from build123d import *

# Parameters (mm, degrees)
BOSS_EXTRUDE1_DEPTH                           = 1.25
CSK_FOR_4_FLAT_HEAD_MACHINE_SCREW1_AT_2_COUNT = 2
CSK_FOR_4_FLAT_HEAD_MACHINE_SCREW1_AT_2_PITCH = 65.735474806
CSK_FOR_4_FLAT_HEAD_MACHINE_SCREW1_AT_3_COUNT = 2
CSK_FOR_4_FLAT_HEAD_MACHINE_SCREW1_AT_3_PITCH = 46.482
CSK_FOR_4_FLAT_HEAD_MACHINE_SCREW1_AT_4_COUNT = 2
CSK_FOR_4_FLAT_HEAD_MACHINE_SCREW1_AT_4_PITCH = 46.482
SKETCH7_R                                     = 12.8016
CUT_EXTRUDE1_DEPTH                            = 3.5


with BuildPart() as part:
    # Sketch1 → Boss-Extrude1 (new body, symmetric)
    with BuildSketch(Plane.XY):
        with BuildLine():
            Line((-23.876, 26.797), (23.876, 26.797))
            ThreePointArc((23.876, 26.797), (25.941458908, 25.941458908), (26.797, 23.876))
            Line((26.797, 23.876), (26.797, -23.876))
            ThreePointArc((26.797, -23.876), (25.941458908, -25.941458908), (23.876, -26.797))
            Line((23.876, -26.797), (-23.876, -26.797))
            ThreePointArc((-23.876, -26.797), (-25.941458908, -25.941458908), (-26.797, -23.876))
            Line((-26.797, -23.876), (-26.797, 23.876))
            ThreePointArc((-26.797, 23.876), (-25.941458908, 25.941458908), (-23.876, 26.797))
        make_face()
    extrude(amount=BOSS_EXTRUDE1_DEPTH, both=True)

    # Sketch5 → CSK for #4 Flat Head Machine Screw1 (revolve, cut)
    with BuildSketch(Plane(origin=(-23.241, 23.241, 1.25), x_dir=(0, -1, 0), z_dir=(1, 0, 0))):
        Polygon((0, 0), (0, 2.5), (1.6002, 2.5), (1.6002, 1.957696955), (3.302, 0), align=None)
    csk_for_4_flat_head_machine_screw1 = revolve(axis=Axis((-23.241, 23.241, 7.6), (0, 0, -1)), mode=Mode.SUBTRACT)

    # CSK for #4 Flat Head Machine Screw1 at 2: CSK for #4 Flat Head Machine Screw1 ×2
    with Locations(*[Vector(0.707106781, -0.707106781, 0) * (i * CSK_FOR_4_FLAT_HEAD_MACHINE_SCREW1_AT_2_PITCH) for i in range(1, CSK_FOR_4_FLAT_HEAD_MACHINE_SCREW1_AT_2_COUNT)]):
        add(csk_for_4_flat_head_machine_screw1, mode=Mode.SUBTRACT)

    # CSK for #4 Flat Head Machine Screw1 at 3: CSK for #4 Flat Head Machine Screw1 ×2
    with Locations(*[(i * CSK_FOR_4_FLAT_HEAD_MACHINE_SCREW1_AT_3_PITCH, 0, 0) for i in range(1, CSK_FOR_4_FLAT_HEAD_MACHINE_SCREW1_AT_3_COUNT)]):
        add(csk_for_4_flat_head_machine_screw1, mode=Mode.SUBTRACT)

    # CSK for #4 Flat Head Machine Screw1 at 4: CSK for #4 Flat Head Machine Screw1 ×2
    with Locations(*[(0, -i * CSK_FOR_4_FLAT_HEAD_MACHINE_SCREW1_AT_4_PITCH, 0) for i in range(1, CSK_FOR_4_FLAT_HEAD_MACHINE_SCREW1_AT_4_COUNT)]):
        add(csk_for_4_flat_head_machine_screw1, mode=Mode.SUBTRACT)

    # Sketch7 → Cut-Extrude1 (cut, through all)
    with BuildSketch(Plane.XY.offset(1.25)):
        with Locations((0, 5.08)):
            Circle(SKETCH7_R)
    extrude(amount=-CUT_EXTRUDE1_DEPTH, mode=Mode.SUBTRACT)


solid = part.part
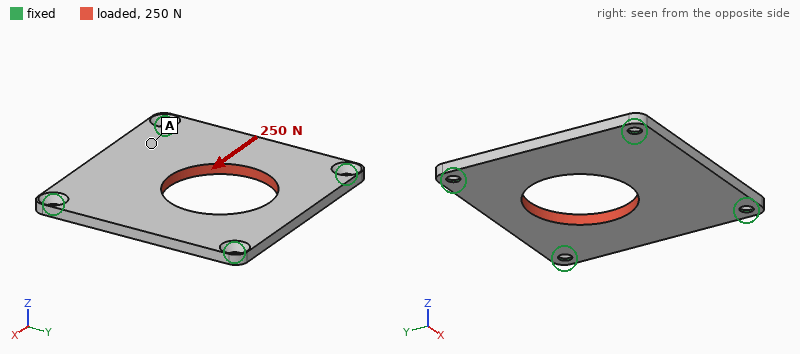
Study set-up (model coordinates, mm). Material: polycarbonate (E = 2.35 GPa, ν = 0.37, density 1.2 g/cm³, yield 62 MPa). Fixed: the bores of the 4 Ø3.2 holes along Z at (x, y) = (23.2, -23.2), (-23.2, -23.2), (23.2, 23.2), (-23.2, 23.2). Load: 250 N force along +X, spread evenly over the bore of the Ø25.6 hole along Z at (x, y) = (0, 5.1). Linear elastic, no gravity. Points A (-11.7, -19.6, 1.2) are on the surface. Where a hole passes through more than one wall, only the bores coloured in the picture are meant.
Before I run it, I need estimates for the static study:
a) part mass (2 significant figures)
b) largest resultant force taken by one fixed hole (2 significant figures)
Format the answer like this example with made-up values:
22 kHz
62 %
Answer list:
6.8 g
68 N
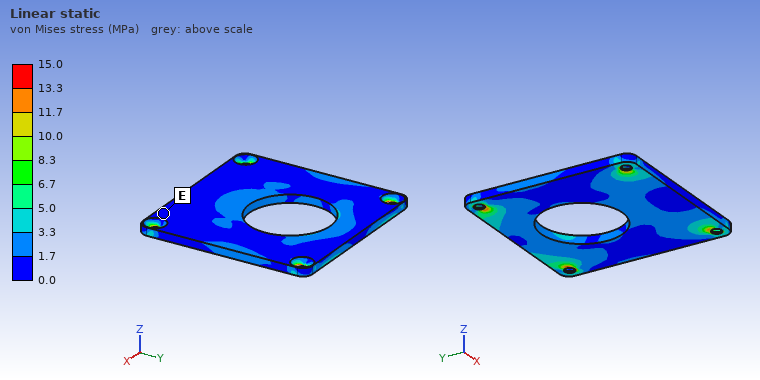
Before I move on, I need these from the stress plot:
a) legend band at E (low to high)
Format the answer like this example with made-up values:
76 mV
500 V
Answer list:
0.0 to 1.7 MPa
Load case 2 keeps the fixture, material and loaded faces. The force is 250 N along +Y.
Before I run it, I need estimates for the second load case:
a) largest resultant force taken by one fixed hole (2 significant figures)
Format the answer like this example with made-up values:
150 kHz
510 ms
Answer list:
66 N
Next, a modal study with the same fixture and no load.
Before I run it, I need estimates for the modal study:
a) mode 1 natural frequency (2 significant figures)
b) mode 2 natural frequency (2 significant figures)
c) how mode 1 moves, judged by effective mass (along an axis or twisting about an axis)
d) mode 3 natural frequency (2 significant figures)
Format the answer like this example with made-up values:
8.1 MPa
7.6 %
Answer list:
960 Hz
1500 Hz
along Z
1500 Hz
